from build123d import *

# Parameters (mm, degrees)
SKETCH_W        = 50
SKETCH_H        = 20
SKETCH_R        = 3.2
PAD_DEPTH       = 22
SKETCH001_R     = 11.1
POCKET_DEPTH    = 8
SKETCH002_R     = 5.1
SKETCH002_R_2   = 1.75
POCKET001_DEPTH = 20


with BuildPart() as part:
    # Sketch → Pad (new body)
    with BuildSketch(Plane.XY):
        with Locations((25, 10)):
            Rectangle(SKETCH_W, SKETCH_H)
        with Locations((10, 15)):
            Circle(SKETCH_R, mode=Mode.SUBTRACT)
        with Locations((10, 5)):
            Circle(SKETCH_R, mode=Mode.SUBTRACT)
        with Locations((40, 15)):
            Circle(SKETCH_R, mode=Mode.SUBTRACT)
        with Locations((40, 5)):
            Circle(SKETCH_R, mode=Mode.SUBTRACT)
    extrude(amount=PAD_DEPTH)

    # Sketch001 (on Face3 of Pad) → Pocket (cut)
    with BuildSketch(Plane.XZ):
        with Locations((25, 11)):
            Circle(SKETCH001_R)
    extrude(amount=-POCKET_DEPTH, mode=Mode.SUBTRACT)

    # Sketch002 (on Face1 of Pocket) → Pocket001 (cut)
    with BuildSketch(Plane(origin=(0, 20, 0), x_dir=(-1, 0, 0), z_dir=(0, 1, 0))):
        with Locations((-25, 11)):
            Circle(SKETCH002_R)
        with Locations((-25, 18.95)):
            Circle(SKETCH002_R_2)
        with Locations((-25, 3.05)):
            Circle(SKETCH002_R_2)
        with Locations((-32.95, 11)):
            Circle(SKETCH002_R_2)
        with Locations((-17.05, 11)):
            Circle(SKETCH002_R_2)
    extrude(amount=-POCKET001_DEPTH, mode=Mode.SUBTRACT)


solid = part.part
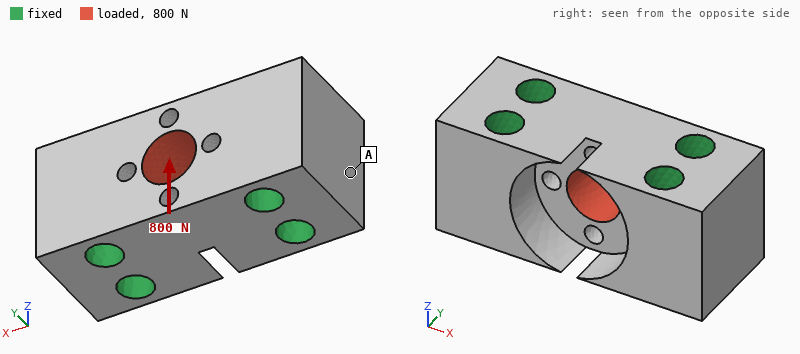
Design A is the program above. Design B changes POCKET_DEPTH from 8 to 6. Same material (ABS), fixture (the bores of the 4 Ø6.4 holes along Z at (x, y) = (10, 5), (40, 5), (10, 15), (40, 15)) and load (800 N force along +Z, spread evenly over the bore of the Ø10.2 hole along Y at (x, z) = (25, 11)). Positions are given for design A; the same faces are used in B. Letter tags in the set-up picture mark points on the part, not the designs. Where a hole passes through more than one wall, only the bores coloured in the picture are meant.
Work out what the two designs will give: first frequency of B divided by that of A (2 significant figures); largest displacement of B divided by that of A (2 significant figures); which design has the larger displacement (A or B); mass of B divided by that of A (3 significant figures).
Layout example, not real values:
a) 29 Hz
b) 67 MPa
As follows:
a) 1.00
b) 0.86
c) A
d) 1.04
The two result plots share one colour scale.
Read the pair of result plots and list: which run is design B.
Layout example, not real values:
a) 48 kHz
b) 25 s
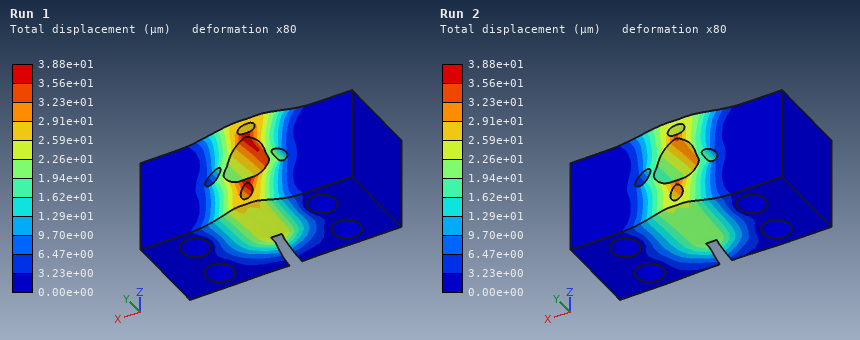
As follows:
a) Run 2
